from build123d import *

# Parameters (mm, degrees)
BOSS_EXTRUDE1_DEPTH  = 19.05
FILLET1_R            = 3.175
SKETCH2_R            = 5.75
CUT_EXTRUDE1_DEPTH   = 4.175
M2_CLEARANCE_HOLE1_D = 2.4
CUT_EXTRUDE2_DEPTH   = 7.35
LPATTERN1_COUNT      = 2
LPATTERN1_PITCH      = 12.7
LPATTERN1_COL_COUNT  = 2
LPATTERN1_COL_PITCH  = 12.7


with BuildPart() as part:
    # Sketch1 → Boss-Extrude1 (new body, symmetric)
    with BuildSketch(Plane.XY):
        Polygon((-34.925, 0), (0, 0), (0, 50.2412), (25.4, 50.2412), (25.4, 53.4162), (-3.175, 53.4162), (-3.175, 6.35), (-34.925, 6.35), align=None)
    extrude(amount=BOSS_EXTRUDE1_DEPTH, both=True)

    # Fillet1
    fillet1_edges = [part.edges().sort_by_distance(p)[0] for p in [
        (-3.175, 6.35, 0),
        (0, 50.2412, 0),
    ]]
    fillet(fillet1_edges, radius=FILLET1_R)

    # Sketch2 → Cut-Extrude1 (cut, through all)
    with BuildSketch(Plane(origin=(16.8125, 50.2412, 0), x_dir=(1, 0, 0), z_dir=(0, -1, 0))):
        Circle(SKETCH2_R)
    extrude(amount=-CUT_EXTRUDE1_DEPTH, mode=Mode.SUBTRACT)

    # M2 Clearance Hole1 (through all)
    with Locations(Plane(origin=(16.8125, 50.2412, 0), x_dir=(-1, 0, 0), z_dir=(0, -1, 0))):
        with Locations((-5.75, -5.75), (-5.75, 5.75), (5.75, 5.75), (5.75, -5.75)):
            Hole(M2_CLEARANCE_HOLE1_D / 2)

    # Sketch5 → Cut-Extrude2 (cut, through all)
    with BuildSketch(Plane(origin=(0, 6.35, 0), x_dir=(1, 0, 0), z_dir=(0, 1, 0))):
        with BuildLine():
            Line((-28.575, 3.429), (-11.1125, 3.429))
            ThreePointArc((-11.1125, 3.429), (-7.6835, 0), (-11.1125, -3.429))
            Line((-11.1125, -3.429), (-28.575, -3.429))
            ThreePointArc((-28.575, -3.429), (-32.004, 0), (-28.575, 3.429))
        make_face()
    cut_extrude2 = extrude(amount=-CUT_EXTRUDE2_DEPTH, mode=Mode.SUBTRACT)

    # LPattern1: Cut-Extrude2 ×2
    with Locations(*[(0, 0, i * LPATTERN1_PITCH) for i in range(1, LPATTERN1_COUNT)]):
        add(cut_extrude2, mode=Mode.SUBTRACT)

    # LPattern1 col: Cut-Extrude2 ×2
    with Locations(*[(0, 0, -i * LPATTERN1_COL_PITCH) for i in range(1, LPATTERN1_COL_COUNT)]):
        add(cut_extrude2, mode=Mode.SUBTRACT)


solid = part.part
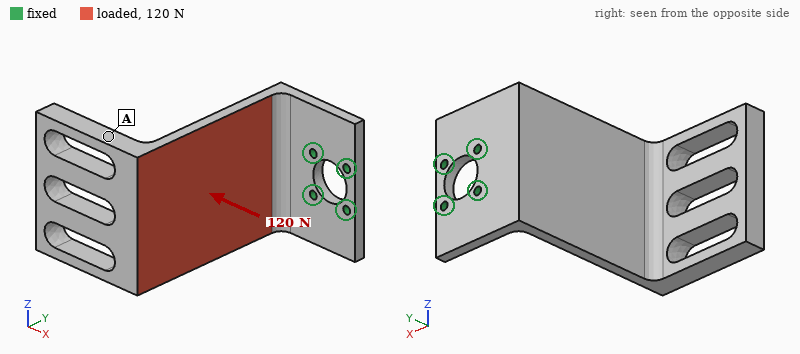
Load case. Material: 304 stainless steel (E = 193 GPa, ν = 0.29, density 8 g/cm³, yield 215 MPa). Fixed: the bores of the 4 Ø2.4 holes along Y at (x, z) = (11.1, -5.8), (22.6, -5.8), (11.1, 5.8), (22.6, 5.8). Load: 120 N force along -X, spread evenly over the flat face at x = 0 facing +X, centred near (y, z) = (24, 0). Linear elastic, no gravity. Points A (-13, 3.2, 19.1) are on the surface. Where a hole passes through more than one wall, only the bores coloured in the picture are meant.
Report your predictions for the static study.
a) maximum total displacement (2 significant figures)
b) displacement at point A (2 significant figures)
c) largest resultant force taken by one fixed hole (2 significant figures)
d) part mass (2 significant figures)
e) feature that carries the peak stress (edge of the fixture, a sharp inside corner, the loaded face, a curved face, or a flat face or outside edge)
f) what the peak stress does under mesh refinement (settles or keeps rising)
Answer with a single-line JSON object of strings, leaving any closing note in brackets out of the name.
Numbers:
{"maximum total displacement": "0.26 mm", "displacement at point A": "0.20 mm", "largest resultant force taken by one fixed hole": "78 N", "part mass": "110 g", "feature that carries the peak stress": "edge of the fixture", "what the peak stress does under mesh refinement": "keeps rising"}
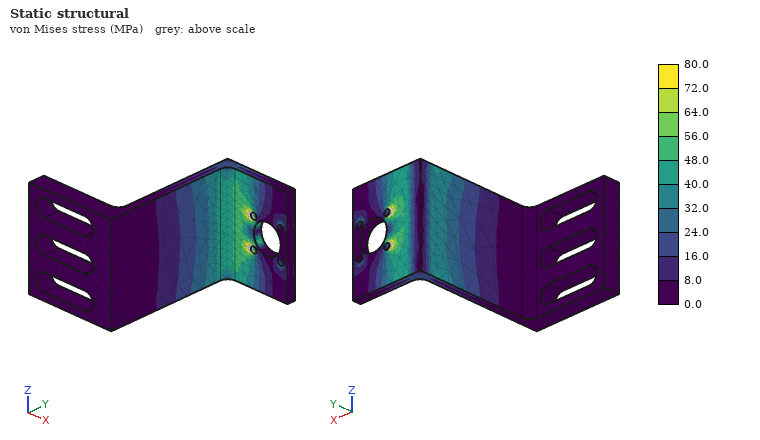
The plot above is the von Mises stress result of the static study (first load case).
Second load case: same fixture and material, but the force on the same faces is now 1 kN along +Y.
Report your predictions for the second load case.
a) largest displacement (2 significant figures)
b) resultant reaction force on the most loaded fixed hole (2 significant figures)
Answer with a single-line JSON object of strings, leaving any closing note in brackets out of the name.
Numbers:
{"largest displacement": "0.16 mm", "resultant reaction force on the most loaded fixed hole": "640 N"}
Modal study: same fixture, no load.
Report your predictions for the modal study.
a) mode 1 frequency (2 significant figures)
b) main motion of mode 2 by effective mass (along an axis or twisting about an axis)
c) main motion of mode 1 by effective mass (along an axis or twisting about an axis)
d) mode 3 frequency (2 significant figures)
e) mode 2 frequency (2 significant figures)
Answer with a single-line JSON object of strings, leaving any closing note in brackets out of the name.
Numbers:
{"mode 1 frequency": "350 Hz", "main motion of mode 2 by effective mass": "along Z", "main motion of mode 1 by effective mass": "along X", "mode 3 frequency": "1300 Hz", "mode 2 frequency": "880 Hz"}
